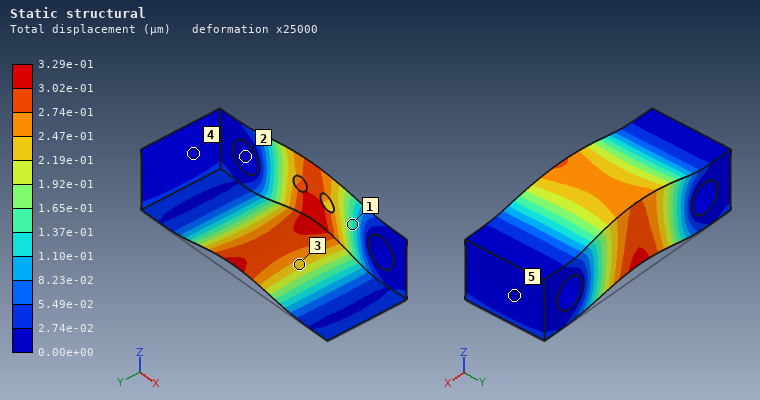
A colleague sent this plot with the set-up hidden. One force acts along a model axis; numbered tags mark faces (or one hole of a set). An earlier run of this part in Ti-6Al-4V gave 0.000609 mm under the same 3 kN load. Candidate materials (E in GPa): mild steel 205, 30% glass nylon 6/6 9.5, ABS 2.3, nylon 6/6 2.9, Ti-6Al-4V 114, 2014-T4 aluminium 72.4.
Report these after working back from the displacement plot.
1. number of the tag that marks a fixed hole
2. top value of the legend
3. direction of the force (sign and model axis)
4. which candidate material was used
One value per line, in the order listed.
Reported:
2
3.29e-01 µm
+Z
mild steel
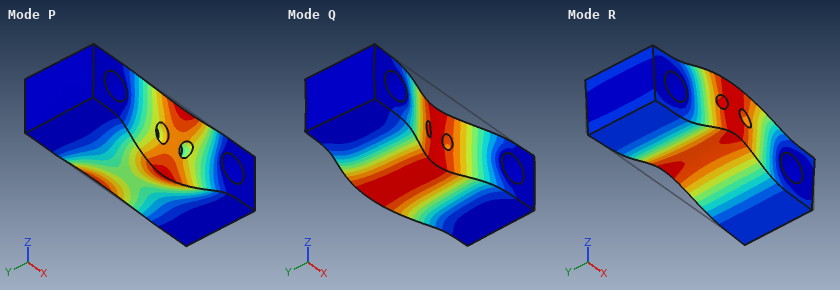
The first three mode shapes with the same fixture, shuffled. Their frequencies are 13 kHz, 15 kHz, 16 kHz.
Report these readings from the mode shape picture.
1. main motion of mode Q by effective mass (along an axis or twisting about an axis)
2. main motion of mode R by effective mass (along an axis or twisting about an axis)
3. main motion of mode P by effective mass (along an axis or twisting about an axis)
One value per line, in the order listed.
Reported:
along Y
along Z
twisting about X
